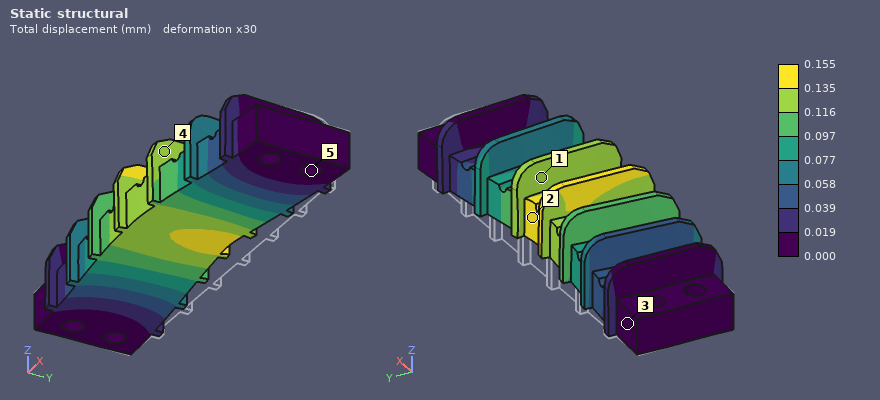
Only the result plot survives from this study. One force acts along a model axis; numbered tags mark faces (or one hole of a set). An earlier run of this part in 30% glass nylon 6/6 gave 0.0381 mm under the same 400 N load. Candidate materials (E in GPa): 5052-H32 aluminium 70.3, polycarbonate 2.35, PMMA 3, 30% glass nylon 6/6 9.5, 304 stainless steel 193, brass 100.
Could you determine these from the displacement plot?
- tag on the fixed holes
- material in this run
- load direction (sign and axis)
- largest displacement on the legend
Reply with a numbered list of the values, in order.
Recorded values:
1. 5
2. polycarbonate
3. -Y
4. 0.155 mm
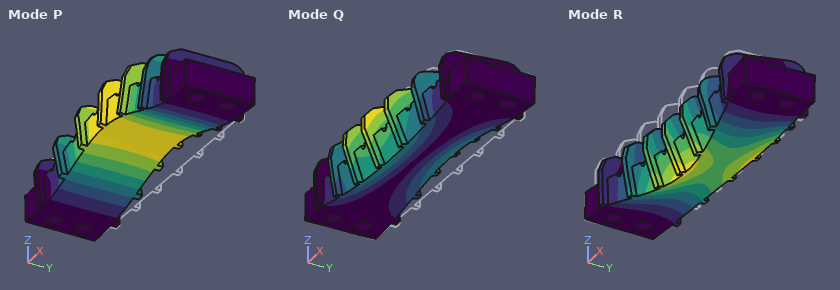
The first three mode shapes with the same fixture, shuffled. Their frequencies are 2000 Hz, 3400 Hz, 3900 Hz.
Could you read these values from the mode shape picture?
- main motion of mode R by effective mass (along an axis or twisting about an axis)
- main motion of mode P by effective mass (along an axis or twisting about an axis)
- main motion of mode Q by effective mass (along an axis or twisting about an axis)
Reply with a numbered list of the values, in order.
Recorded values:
1. along Y
2. along Z
3. along Y
